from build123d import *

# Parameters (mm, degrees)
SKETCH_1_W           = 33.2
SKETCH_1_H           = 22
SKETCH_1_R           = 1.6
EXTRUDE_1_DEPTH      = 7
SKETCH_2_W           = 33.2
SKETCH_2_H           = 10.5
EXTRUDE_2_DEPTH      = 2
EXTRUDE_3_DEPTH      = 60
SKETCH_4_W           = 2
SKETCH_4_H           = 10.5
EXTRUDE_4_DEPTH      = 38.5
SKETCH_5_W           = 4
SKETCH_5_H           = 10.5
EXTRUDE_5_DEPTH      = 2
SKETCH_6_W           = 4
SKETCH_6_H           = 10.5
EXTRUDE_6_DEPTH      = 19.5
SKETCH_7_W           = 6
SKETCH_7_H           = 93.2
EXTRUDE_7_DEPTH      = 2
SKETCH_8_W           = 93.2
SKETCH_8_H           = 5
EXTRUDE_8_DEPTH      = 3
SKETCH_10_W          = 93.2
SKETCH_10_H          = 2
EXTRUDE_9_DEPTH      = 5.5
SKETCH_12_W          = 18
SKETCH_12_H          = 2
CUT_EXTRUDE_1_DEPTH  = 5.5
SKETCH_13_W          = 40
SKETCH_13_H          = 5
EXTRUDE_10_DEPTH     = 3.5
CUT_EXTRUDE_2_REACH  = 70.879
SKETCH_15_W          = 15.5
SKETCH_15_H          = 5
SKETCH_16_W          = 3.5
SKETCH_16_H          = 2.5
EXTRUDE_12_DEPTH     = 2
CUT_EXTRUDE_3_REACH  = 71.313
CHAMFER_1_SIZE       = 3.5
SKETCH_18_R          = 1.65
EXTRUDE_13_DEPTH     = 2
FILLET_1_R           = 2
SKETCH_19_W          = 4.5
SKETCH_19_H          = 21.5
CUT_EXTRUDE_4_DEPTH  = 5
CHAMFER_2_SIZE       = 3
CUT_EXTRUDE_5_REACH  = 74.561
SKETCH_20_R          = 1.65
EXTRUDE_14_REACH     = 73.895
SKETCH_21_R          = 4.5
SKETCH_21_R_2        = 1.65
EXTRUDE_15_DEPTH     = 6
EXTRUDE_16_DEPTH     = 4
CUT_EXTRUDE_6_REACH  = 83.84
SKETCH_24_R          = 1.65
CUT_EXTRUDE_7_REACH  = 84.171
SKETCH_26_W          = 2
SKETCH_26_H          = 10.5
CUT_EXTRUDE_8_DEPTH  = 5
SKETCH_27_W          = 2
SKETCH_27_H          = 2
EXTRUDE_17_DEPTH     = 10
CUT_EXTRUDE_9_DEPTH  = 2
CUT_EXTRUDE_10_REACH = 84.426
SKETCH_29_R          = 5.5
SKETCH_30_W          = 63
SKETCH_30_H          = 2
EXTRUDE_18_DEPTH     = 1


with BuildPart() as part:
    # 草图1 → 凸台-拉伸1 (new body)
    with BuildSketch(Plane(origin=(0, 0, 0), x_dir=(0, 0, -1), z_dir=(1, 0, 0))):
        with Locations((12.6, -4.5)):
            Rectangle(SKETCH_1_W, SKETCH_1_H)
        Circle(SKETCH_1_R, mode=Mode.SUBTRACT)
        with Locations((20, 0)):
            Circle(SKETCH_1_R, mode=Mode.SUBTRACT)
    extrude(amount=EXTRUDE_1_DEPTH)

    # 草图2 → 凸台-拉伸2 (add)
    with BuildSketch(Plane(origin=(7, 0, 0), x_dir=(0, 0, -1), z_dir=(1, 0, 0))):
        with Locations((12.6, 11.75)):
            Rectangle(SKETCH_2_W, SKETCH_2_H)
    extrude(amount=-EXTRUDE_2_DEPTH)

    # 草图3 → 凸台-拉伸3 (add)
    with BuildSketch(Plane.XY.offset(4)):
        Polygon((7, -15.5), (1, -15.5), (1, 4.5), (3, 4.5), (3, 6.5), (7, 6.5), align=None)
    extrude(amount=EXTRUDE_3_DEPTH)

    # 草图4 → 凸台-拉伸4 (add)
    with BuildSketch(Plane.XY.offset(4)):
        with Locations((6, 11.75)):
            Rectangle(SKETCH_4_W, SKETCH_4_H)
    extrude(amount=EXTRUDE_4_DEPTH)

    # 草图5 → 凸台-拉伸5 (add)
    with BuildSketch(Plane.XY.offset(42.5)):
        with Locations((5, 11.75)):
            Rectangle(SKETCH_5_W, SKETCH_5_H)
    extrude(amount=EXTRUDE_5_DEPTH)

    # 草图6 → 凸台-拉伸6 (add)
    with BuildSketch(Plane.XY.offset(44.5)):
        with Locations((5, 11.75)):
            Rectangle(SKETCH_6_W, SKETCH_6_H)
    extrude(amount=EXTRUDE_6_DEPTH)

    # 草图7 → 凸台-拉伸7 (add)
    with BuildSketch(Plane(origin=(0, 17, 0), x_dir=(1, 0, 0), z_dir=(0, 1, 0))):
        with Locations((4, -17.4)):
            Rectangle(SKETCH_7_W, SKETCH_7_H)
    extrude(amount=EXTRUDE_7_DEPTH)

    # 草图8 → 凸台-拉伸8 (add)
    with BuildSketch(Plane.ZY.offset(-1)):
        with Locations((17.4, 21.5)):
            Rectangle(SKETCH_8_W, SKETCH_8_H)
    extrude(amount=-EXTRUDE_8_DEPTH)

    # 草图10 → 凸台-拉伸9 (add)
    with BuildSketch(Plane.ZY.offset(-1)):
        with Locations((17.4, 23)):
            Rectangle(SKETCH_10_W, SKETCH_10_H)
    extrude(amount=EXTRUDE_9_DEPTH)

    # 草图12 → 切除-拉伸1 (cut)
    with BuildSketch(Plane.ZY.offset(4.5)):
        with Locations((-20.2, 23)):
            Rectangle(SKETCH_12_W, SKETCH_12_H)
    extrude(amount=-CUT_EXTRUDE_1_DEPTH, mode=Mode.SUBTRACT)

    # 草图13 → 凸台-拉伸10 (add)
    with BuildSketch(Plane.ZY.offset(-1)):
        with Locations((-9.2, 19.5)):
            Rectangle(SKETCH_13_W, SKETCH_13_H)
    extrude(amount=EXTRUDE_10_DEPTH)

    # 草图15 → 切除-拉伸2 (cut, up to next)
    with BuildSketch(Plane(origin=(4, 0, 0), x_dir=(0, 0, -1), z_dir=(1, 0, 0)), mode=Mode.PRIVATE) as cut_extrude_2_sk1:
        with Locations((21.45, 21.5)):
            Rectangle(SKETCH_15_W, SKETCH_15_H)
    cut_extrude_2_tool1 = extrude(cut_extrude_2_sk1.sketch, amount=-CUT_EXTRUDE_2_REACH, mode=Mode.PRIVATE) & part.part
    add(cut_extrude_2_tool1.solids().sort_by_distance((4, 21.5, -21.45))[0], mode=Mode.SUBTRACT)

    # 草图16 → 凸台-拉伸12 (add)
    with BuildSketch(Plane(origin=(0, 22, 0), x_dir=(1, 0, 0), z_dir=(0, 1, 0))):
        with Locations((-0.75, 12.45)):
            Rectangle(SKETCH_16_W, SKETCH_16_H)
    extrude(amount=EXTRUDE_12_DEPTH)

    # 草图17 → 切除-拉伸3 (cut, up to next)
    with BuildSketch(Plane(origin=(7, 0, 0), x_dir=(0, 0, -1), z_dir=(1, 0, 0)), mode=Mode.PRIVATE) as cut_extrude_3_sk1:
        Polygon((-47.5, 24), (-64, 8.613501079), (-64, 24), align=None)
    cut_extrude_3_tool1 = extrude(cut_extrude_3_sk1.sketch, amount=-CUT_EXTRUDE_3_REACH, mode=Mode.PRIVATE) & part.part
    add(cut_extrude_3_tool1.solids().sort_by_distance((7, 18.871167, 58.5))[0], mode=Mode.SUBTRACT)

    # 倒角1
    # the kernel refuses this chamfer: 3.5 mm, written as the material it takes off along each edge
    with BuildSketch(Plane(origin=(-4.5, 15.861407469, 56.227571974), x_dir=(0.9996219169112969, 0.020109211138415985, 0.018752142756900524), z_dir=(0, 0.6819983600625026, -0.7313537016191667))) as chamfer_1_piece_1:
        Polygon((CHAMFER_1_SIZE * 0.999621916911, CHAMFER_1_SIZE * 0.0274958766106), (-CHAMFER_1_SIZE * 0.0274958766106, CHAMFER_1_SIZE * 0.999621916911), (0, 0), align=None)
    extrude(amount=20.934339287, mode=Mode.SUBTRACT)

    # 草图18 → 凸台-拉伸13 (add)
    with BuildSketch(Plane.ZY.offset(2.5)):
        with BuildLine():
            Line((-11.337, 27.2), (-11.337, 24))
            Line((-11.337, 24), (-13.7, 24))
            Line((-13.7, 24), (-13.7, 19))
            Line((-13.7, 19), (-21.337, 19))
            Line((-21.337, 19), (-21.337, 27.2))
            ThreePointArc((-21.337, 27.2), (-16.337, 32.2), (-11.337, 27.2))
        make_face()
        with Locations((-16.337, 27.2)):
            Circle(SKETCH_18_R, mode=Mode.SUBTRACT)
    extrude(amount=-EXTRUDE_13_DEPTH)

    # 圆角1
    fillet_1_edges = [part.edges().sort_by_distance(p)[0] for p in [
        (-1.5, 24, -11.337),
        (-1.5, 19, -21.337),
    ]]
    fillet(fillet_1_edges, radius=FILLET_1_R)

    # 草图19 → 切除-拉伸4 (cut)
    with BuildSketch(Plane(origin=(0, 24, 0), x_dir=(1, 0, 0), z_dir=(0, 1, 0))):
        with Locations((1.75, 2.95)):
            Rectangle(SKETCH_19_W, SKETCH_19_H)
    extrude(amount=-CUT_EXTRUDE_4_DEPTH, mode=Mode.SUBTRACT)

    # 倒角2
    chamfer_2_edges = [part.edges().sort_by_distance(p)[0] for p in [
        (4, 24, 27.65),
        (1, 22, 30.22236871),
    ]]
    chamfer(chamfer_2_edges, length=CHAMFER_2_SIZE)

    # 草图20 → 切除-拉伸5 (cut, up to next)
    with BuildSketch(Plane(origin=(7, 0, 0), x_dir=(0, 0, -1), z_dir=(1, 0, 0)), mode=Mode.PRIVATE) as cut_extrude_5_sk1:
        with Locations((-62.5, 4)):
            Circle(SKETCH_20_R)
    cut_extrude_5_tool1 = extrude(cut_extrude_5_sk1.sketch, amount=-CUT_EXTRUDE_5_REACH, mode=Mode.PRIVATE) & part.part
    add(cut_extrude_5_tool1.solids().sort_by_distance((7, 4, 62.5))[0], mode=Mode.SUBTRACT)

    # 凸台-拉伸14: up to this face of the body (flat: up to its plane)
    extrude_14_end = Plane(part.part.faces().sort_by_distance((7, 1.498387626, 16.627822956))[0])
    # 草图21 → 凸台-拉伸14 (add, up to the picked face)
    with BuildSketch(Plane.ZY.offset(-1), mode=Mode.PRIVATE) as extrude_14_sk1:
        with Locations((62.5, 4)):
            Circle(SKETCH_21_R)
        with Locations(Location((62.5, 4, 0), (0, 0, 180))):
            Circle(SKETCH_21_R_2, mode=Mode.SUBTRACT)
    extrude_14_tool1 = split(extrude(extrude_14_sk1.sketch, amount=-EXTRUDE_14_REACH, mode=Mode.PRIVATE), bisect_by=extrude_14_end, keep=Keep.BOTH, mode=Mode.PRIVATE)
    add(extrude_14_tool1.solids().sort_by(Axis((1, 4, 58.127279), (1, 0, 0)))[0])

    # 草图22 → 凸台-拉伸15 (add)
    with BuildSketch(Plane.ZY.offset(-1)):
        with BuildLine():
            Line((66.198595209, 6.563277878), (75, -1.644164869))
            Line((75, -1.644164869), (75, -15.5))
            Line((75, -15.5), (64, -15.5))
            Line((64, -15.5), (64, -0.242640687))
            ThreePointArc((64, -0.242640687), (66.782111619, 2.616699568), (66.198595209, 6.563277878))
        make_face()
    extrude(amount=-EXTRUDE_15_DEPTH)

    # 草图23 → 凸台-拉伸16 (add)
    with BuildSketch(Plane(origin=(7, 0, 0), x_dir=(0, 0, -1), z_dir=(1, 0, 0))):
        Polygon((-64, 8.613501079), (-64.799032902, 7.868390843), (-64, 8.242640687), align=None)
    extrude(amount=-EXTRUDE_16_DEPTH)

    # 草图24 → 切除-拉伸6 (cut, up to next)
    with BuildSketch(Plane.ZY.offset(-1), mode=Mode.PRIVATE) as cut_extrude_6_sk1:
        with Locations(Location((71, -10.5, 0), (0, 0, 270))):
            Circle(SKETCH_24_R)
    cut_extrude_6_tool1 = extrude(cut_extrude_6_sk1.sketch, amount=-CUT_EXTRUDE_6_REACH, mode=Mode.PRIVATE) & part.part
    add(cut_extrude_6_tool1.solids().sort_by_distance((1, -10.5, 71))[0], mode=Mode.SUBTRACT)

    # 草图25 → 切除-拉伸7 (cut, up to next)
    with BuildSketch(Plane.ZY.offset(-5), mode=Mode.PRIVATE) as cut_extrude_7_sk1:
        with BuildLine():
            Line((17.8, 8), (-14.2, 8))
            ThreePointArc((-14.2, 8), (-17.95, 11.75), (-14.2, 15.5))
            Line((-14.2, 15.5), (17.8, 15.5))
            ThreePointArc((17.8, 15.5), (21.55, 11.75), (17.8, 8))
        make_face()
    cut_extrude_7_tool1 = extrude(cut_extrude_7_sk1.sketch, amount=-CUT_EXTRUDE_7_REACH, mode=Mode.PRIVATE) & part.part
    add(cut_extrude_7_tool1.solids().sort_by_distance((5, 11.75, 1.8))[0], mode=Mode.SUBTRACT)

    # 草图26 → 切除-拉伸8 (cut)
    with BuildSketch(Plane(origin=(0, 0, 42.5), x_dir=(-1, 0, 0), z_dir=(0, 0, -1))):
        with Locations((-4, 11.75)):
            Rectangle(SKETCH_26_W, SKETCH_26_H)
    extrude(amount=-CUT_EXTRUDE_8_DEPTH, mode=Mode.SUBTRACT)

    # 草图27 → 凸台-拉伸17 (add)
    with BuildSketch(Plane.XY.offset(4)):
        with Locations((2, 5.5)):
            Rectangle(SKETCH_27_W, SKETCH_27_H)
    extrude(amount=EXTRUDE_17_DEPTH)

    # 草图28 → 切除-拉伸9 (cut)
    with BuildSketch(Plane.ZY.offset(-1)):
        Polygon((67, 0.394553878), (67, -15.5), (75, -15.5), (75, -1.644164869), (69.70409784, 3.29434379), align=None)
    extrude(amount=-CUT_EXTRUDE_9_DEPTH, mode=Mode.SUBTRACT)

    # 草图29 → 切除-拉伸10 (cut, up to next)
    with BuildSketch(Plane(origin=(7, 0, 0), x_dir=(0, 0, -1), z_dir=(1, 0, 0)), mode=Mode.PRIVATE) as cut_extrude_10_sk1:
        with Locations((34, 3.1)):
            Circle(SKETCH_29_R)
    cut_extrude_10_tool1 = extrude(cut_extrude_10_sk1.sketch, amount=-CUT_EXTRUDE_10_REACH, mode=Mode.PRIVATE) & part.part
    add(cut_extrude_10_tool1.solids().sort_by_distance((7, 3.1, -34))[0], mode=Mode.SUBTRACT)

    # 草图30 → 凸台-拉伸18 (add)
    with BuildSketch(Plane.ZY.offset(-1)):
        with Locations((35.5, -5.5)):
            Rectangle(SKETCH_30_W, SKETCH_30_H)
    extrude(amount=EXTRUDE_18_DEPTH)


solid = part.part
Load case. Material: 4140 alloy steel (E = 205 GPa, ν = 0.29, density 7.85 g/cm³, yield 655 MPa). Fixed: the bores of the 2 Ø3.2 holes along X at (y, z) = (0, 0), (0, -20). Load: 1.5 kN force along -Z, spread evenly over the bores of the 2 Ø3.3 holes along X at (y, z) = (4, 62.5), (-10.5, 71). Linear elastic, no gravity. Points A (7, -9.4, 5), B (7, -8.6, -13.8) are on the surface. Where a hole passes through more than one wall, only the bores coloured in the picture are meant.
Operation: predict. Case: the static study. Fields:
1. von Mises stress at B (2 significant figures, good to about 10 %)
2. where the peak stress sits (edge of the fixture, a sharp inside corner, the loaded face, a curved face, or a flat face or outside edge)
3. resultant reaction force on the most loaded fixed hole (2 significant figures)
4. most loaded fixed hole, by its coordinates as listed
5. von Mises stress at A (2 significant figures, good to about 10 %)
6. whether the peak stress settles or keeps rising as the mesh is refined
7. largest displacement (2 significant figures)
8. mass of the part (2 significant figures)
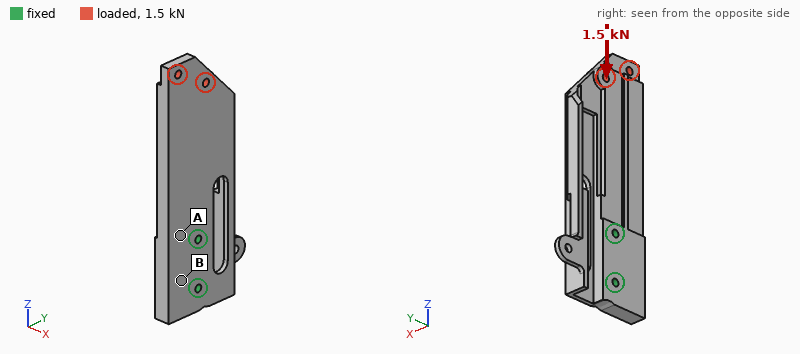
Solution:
4.1 MPa
edge of the fixture
1.1 kN
(0, 0)
10 MPa
keeps rising
15 µm
140 g
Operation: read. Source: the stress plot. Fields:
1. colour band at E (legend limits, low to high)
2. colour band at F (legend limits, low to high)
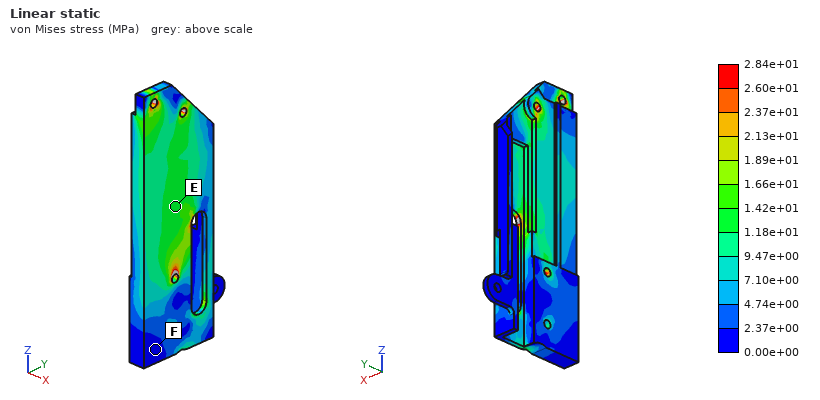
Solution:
1.18e+01 to 1.42e+01 MPa
0.00e+00 to 2.37e+00 MPa
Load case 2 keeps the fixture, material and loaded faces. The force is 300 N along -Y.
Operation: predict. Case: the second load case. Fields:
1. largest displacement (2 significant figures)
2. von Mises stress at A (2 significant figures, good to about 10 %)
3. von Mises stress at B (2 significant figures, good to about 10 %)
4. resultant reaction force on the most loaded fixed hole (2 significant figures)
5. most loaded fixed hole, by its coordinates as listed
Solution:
31 µm
14 MPa
10 MPa
1.1 kN
(0, 0)
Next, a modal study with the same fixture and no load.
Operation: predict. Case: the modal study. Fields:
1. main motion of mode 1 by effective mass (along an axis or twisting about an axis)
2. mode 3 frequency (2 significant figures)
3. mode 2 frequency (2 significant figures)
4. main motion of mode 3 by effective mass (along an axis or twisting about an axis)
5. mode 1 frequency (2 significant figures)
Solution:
along X
2800 Hz
1900 Hz
along Y
1000 Hz
